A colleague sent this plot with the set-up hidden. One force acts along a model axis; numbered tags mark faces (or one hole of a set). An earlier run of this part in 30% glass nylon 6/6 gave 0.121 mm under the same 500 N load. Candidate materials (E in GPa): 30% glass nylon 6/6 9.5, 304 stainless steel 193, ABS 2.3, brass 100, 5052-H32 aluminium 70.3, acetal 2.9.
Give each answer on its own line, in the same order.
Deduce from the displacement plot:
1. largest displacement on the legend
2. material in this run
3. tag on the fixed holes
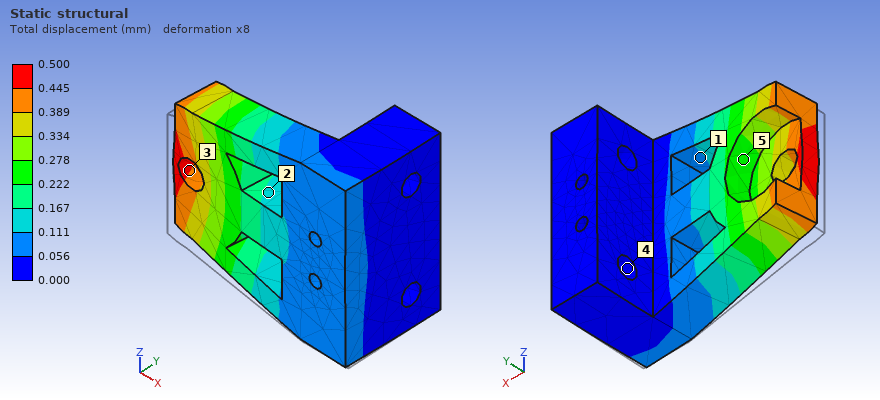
0.500 mm
ABS
4
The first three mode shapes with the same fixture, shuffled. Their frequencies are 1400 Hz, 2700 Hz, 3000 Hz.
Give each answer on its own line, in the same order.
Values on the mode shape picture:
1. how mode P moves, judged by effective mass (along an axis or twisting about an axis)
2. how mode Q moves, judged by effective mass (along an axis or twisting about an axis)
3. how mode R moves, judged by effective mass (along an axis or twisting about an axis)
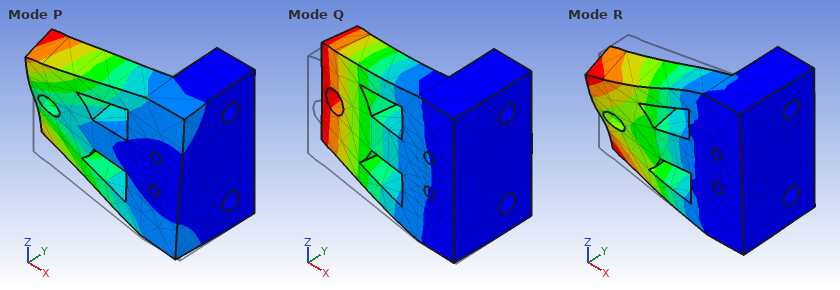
along Z
along Y
along Z
